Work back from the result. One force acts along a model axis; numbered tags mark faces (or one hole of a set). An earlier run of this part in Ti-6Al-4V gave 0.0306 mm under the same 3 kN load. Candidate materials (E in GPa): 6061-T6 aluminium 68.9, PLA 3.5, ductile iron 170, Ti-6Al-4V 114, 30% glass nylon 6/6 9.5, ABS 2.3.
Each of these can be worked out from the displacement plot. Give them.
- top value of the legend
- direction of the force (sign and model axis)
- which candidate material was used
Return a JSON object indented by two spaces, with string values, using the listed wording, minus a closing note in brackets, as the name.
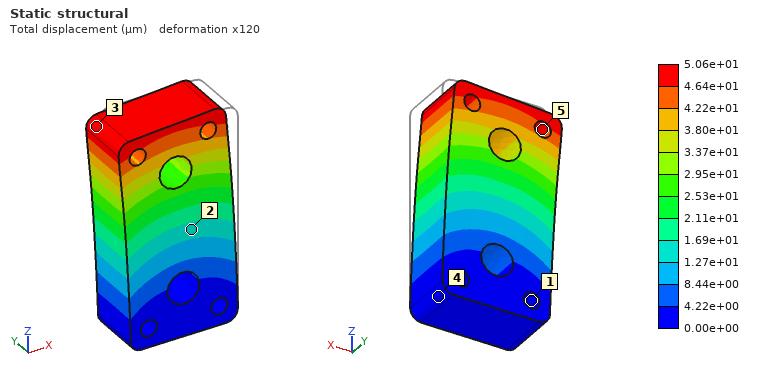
{
  "top value of the legend": "5.06e+01 µm",
  "direction of the force": "-X",
  "which candidate material was used": "6061-T6 aluminium"
}
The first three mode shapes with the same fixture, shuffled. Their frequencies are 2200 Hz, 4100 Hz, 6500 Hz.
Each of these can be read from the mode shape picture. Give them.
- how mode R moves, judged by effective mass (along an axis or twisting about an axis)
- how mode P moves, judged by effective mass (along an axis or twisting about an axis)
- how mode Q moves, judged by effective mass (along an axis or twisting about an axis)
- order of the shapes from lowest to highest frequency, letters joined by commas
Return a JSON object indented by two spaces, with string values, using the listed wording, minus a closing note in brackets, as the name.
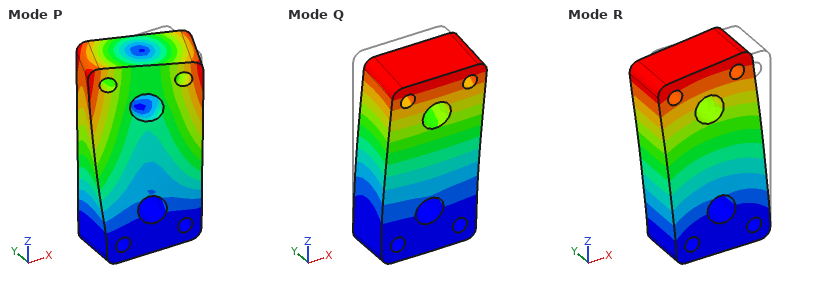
{
  "how mode R moves, judged by effective mass": "along X",
  "how mode P moves, judged by effective mass": "twisting about Z",
  "how mode Q moves, judged by effective mass": "along Y",
  "order of the shapes from lowest to highest frequency, letters joined by commas": "Q, R, P"
}
